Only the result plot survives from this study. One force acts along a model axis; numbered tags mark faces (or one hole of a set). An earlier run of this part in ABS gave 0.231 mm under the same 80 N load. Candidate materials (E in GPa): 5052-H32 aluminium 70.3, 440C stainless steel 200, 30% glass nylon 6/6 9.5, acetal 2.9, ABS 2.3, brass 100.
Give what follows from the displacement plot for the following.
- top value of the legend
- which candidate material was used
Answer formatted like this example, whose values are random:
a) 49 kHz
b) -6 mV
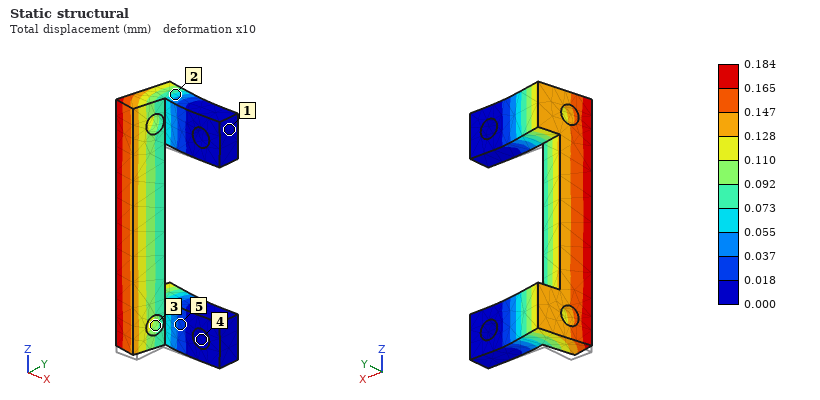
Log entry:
a) 0.184 mm
b) acetal
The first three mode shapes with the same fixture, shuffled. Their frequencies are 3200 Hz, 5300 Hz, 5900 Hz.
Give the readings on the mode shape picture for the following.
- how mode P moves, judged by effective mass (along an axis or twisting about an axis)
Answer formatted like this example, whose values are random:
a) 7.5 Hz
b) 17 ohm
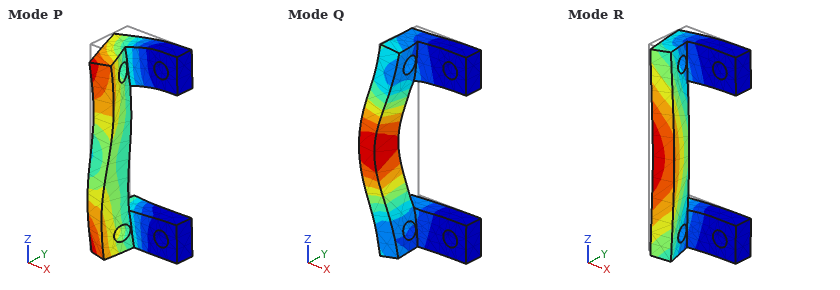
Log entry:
a) along Z
